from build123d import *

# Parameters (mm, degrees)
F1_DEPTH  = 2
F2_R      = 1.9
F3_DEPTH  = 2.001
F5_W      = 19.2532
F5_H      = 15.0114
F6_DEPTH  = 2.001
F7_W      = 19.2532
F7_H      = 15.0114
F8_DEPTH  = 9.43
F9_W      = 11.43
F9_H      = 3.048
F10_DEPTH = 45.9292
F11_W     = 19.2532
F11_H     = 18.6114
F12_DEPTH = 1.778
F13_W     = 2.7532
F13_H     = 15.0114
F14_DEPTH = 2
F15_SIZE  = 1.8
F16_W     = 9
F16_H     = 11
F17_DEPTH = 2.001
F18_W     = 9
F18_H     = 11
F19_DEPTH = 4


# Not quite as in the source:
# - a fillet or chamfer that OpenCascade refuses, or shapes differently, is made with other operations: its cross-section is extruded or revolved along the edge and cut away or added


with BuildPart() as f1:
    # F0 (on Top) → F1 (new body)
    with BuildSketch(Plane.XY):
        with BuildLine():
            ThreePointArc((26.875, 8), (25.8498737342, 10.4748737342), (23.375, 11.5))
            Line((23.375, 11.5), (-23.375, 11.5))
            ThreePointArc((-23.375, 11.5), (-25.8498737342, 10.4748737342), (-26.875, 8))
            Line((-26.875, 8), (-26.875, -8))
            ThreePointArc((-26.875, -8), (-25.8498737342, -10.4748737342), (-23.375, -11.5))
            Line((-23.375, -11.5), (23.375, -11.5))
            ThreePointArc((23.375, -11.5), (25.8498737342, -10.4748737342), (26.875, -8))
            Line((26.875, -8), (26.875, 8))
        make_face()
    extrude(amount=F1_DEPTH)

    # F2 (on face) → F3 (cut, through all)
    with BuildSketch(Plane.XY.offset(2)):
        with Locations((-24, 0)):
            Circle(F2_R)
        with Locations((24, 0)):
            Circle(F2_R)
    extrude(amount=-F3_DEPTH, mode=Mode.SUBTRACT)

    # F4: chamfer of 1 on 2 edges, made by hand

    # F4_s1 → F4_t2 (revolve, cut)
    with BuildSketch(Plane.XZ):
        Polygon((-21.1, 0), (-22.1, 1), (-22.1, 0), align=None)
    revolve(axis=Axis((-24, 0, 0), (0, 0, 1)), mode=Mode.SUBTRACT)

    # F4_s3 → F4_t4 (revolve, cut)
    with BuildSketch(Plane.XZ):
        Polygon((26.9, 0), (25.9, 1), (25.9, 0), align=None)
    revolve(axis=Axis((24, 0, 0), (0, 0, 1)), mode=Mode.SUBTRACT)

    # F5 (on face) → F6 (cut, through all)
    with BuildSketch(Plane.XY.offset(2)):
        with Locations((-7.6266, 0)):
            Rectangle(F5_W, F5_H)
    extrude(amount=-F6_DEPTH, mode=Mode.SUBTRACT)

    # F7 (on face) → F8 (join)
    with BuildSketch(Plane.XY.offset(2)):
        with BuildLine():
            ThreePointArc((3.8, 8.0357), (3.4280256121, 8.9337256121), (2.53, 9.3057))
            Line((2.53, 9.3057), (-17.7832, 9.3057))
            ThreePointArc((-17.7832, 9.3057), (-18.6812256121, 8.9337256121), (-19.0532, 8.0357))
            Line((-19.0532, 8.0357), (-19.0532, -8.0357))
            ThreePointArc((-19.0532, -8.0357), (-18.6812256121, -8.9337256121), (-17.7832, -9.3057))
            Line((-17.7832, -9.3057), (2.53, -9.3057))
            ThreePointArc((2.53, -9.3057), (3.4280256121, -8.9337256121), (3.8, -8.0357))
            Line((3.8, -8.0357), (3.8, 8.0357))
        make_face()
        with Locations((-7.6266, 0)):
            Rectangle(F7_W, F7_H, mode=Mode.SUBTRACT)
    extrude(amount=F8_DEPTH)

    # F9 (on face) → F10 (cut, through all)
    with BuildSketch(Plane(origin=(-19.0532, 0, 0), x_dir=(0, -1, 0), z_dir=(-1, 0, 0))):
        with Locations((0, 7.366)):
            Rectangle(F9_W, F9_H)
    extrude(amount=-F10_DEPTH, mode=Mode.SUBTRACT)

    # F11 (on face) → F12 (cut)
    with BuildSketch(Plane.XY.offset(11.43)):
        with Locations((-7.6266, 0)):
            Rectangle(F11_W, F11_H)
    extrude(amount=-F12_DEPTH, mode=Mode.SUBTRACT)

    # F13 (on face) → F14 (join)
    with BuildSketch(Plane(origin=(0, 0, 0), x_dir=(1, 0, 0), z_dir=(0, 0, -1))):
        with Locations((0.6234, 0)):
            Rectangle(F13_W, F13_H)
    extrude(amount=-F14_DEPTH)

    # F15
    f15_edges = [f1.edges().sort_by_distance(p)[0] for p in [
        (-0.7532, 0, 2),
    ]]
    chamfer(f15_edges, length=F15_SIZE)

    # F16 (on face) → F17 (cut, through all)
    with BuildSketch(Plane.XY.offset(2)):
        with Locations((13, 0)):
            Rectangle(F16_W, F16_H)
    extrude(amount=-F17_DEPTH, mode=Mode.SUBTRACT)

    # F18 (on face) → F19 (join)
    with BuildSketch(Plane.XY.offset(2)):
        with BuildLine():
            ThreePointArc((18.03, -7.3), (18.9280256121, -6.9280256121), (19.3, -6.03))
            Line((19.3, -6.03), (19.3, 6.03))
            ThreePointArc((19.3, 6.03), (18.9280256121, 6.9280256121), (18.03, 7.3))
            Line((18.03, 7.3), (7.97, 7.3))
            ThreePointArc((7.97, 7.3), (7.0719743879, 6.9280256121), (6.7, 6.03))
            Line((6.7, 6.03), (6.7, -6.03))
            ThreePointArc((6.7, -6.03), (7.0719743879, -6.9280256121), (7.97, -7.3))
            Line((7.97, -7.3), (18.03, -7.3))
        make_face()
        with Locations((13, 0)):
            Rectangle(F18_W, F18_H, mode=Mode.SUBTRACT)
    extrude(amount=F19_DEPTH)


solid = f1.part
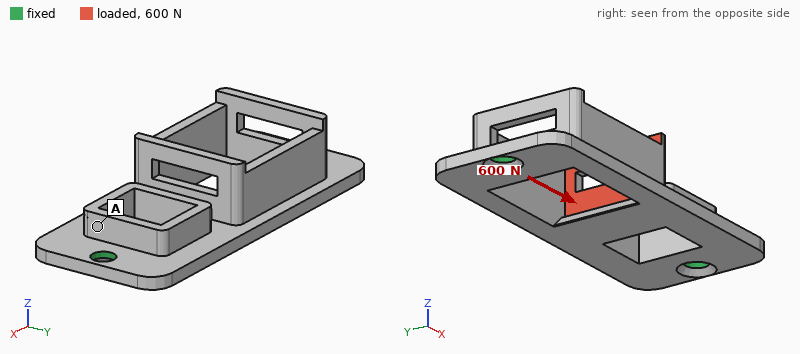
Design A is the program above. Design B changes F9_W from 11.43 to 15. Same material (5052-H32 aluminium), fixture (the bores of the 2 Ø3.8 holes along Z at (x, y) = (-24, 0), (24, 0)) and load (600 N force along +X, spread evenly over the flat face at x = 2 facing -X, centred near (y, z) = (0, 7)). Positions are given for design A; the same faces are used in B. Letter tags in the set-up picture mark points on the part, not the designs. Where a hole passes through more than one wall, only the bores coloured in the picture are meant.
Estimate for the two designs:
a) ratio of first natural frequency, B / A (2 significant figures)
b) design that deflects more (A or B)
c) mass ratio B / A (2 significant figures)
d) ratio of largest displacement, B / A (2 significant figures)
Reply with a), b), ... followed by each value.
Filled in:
a) 1.0
b) B
c) 0.99
d) 1.2
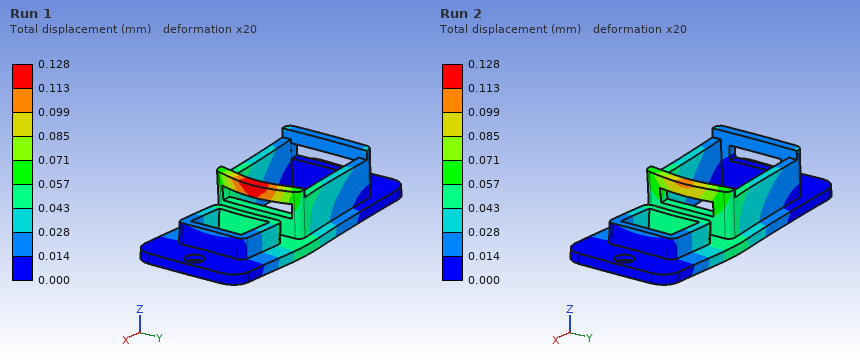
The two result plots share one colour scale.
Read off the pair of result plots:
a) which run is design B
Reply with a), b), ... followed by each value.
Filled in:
a) Run 1
